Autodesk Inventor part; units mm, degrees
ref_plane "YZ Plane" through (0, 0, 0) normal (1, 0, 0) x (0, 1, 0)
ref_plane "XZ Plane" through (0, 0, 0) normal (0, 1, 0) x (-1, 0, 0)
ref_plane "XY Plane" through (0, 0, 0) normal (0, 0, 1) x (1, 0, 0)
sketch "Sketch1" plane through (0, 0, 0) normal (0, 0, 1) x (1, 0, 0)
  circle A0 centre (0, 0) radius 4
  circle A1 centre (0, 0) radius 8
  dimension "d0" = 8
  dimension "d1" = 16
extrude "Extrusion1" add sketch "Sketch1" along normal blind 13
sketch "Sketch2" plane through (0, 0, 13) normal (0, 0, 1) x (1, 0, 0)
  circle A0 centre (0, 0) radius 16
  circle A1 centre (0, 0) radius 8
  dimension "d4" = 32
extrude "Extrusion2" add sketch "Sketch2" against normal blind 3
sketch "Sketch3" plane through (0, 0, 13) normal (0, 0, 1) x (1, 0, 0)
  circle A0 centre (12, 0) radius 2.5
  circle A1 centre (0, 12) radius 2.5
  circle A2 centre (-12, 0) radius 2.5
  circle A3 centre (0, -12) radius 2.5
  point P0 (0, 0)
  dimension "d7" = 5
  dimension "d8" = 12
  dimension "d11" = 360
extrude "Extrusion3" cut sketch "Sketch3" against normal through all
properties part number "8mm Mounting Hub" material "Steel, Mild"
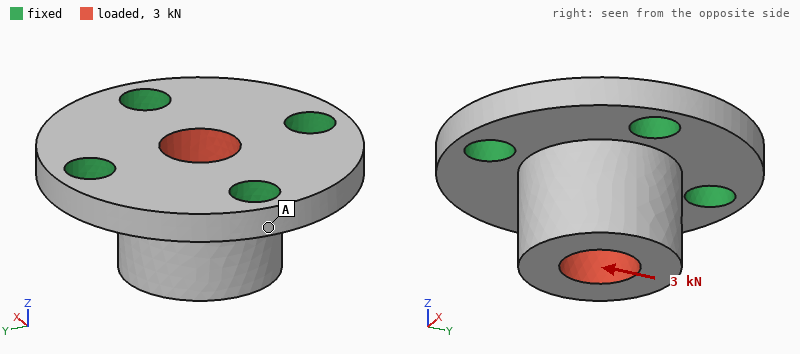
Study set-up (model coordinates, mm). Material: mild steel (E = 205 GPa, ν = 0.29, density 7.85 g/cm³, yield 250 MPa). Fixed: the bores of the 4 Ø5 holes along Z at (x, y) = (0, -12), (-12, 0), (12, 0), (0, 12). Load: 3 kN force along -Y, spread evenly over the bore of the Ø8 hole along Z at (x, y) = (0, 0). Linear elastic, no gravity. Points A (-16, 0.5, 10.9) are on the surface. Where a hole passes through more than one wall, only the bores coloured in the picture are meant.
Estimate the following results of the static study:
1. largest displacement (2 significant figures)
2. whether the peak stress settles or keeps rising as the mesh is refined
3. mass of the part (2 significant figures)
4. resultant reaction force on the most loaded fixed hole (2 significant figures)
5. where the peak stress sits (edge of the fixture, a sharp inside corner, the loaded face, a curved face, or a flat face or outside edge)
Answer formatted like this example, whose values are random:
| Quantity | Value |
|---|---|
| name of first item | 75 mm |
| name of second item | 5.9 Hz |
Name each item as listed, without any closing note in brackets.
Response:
| Quantity | Value |
|---|---|
| largest displacement | 5.5 µm |
| whether the peak stress settles or keeps rising as the mesh is refined | keeps rising |
| mass of the part | 28 g |
| resultant reaction force on the most loaded fixed hole | 1.2 kN |
| where the peak stress sits | edge of the fixture |
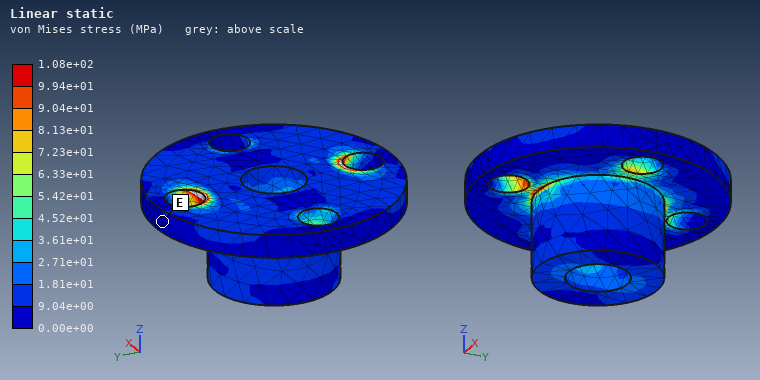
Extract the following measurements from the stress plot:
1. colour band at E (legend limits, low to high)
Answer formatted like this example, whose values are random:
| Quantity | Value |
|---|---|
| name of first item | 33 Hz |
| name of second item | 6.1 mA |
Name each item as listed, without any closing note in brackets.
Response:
| Quantity | Value |
|---|---|
| colour band at E | 0.00e+00 to 9.04e+00 MPa |
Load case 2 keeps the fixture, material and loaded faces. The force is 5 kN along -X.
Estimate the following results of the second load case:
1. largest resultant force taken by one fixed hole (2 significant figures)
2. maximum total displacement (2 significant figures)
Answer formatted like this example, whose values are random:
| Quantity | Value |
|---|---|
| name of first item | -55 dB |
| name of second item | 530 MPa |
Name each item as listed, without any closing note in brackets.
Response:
| Quantity | Value |
|---|---|
| largest resultant force taken by one fixed hole | 2.1 kN |
| maximum total displacement | 9.1 µm |
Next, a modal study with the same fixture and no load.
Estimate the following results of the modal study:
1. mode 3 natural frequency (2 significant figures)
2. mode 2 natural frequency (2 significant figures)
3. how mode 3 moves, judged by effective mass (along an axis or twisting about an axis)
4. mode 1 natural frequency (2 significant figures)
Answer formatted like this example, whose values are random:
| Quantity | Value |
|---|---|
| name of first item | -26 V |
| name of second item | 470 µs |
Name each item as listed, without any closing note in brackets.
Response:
| Quantity | Value |
|---|---|
| mode 3 natural frequency | 44 kHz |
| mode 2 natural frequency | 34 kHz |
| how mode 3 moves, judged by effective mass | along Z |
| mode 1 natural frequency | 34 kHz |
